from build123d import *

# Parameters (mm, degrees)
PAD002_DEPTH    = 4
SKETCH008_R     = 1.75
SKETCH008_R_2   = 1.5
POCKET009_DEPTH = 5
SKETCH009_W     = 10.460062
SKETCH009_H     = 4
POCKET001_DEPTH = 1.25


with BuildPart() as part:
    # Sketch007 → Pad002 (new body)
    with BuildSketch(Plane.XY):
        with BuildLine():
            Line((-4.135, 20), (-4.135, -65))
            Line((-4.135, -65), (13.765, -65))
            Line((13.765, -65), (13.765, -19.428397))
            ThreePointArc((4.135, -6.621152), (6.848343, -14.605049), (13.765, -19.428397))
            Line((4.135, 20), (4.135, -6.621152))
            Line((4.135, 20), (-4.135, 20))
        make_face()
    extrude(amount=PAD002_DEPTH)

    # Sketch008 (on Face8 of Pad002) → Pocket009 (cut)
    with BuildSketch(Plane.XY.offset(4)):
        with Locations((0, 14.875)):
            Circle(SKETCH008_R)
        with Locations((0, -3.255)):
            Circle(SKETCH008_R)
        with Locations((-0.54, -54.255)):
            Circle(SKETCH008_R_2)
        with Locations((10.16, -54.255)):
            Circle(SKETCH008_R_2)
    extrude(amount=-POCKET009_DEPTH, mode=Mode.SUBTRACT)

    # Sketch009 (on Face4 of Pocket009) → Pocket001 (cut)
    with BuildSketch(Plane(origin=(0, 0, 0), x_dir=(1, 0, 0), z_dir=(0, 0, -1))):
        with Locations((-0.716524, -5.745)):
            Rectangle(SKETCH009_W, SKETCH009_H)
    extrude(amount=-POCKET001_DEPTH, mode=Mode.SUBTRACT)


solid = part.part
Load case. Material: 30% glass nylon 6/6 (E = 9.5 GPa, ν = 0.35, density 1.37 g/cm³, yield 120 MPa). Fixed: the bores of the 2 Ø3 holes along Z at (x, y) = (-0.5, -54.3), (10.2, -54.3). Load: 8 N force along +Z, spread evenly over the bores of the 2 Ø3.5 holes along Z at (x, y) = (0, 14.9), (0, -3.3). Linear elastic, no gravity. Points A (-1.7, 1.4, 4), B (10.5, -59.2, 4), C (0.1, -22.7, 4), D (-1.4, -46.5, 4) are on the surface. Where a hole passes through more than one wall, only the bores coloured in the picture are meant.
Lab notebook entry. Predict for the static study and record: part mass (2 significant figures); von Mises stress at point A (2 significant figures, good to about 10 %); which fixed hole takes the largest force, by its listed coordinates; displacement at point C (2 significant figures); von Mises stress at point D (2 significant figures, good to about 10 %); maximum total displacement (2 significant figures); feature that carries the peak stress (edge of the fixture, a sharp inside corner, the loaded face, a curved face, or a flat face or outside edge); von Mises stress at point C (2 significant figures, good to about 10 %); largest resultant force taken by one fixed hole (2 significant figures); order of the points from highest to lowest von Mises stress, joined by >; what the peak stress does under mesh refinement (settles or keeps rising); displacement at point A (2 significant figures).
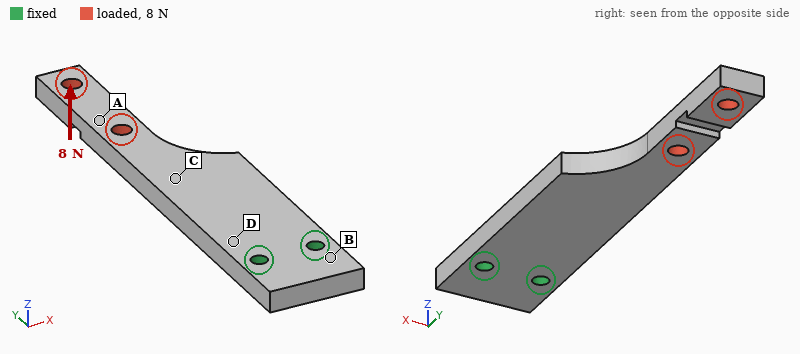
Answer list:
6.2 g
2.7 MPa
(-0.5, -54.3)
0.21 mm
8.8 MPa
0.98 mm
edge of the fixture
5.7 MPa
6.9 N
D > C > A > B
keeps rising
0.60 mm
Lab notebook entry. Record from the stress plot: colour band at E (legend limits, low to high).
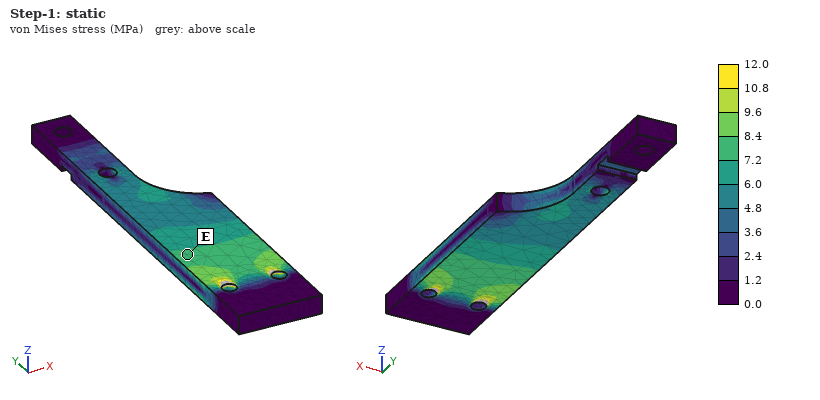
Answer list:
7.2 to 8.4 MPa
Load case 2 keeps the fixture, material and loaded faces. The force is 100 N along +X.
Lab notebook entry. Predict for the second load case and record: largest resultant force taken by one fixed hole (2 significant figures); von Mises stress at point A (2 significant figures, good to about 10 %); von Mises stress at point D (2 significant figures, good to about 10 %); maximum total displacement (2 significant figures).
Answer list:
500 N
8.9 MPa
17 MPa
0.97 mm
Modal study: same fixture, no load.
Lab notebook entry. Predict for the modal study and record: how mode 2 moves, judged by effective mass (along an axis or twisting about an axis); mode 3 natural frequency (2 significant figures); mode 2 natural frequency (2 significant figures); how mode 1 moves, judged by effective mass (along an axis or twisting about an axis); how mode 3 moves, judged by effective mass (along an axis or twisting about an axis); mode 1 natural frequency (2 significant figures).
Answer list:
along X
1900 Hz
1700 Hz
along Z
along Z
450 Hz
